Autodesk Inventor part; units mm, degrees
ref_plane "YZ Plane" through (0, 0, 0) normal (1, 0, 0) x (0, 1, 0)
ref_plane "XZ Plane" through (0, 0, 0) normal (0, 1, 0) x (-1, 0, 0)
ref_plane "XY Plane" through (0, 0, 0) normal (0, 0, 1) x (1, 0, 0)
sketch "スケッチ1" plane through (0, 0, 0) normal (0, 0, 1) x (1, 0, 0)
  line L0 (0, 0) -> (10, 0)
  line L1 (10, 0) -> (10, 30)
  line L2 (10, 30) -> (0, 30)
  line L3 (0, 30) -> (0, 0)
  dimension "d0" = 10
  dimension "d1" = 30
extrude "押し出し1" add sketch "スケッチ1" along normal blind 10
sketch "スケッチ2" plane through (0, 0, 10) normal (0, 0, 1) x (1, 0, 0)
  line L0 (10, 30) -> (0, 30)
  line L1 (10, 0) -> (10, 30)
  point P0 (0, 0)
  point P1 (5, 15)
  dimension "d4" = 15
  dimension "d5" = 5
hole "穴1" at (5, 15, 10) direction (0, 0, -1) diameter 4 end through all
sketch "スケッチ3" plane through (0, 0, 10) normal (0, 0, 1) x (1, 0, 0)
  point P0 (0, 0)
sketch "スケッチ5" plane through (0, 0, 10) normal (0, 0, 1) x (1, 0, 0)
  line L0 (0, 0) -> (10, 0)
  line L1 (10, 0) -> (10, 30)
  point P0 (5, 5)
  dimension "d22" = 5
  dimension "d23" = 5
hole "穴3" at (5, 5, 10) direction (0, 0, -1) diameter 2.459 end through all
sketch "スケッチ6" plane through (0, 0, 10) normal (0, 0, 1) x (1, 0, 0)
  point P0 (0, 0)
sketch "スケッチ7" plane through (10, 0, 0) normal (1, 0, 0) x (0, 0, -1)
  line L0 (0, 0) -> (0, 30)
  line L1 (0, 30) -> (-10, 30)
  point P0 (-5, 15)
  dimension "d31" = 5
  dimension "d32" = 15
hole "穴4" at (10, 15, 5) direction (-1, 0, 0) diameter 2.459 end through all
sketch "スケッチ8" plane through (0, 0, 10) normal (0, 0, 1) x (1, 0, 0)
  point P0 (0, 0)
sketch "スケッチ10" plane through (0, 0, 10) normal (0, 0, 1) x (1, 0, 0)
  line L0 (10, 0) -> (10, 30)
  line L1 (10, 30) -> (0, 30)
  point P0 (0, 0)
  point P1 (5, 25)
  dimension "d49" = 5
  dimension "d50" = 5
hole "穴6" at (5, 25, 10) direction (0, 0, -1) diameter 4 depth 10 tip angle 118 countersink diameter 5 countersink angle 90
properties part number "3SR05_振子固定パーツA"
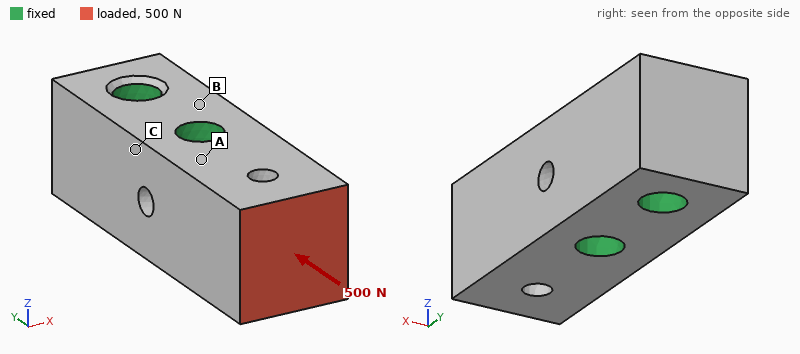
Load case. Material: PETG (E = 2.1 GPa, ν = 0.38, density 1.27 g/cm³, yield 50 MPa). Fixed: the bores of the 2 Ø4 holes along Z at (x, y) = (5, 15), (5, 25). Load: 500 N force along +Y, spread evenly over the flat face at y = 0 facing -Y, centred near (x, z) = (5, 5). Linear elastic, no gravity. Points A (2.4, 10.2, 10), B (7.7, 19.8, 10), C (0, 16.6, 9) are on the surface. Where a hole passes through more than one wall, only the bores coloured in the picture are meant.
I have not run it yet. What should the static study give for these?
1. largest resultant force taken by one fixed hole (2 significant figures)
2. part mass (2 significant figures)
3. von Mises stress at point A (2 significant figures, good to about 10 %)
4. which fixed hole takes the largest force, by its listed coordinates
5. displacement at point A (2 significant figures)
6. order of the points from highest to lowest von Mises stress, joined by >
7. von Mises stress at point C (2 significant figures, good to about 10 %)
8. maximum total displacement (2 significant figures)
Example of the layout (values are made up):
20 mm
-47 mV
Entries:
460 N
3.4 g
5.2 MPa
(5, 15)
13 µm
A > C > B
2.4 MPa
42 µm
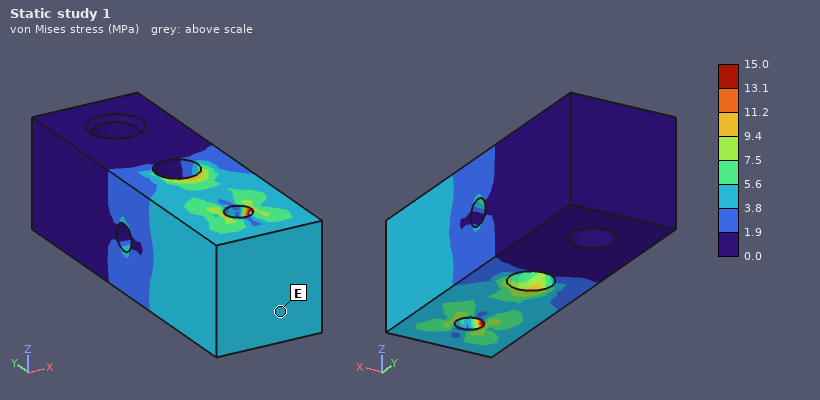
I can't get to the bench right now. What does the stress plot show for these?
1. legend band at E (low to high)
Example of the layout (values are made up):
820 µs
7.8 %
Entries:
3.8 to 5.6 MPa
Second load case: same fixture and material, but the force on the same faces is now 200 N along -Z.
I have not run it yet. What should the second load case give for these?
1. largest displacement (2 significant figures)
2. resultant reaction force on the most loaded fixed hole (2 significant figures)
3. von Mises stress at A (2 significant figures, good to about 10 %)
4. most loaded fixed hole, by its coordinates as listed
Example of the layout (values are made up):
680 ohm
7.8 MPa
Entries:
0.18 mm
220 N
12 MPa
(5, 15)
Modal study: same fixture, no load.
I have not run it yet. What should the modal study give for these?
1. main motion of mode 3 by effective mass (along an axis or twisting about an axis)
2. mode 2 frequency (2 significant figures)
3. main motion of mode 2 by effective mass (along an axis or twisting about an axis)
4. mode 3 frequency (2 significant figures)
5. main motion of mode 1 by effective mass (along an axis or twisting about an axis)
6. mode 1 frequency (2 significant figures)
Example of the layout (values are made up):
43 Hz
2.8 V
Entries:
twisting about Y
7800 Hz
along Z
12 kHz
along X
6300 Hz
